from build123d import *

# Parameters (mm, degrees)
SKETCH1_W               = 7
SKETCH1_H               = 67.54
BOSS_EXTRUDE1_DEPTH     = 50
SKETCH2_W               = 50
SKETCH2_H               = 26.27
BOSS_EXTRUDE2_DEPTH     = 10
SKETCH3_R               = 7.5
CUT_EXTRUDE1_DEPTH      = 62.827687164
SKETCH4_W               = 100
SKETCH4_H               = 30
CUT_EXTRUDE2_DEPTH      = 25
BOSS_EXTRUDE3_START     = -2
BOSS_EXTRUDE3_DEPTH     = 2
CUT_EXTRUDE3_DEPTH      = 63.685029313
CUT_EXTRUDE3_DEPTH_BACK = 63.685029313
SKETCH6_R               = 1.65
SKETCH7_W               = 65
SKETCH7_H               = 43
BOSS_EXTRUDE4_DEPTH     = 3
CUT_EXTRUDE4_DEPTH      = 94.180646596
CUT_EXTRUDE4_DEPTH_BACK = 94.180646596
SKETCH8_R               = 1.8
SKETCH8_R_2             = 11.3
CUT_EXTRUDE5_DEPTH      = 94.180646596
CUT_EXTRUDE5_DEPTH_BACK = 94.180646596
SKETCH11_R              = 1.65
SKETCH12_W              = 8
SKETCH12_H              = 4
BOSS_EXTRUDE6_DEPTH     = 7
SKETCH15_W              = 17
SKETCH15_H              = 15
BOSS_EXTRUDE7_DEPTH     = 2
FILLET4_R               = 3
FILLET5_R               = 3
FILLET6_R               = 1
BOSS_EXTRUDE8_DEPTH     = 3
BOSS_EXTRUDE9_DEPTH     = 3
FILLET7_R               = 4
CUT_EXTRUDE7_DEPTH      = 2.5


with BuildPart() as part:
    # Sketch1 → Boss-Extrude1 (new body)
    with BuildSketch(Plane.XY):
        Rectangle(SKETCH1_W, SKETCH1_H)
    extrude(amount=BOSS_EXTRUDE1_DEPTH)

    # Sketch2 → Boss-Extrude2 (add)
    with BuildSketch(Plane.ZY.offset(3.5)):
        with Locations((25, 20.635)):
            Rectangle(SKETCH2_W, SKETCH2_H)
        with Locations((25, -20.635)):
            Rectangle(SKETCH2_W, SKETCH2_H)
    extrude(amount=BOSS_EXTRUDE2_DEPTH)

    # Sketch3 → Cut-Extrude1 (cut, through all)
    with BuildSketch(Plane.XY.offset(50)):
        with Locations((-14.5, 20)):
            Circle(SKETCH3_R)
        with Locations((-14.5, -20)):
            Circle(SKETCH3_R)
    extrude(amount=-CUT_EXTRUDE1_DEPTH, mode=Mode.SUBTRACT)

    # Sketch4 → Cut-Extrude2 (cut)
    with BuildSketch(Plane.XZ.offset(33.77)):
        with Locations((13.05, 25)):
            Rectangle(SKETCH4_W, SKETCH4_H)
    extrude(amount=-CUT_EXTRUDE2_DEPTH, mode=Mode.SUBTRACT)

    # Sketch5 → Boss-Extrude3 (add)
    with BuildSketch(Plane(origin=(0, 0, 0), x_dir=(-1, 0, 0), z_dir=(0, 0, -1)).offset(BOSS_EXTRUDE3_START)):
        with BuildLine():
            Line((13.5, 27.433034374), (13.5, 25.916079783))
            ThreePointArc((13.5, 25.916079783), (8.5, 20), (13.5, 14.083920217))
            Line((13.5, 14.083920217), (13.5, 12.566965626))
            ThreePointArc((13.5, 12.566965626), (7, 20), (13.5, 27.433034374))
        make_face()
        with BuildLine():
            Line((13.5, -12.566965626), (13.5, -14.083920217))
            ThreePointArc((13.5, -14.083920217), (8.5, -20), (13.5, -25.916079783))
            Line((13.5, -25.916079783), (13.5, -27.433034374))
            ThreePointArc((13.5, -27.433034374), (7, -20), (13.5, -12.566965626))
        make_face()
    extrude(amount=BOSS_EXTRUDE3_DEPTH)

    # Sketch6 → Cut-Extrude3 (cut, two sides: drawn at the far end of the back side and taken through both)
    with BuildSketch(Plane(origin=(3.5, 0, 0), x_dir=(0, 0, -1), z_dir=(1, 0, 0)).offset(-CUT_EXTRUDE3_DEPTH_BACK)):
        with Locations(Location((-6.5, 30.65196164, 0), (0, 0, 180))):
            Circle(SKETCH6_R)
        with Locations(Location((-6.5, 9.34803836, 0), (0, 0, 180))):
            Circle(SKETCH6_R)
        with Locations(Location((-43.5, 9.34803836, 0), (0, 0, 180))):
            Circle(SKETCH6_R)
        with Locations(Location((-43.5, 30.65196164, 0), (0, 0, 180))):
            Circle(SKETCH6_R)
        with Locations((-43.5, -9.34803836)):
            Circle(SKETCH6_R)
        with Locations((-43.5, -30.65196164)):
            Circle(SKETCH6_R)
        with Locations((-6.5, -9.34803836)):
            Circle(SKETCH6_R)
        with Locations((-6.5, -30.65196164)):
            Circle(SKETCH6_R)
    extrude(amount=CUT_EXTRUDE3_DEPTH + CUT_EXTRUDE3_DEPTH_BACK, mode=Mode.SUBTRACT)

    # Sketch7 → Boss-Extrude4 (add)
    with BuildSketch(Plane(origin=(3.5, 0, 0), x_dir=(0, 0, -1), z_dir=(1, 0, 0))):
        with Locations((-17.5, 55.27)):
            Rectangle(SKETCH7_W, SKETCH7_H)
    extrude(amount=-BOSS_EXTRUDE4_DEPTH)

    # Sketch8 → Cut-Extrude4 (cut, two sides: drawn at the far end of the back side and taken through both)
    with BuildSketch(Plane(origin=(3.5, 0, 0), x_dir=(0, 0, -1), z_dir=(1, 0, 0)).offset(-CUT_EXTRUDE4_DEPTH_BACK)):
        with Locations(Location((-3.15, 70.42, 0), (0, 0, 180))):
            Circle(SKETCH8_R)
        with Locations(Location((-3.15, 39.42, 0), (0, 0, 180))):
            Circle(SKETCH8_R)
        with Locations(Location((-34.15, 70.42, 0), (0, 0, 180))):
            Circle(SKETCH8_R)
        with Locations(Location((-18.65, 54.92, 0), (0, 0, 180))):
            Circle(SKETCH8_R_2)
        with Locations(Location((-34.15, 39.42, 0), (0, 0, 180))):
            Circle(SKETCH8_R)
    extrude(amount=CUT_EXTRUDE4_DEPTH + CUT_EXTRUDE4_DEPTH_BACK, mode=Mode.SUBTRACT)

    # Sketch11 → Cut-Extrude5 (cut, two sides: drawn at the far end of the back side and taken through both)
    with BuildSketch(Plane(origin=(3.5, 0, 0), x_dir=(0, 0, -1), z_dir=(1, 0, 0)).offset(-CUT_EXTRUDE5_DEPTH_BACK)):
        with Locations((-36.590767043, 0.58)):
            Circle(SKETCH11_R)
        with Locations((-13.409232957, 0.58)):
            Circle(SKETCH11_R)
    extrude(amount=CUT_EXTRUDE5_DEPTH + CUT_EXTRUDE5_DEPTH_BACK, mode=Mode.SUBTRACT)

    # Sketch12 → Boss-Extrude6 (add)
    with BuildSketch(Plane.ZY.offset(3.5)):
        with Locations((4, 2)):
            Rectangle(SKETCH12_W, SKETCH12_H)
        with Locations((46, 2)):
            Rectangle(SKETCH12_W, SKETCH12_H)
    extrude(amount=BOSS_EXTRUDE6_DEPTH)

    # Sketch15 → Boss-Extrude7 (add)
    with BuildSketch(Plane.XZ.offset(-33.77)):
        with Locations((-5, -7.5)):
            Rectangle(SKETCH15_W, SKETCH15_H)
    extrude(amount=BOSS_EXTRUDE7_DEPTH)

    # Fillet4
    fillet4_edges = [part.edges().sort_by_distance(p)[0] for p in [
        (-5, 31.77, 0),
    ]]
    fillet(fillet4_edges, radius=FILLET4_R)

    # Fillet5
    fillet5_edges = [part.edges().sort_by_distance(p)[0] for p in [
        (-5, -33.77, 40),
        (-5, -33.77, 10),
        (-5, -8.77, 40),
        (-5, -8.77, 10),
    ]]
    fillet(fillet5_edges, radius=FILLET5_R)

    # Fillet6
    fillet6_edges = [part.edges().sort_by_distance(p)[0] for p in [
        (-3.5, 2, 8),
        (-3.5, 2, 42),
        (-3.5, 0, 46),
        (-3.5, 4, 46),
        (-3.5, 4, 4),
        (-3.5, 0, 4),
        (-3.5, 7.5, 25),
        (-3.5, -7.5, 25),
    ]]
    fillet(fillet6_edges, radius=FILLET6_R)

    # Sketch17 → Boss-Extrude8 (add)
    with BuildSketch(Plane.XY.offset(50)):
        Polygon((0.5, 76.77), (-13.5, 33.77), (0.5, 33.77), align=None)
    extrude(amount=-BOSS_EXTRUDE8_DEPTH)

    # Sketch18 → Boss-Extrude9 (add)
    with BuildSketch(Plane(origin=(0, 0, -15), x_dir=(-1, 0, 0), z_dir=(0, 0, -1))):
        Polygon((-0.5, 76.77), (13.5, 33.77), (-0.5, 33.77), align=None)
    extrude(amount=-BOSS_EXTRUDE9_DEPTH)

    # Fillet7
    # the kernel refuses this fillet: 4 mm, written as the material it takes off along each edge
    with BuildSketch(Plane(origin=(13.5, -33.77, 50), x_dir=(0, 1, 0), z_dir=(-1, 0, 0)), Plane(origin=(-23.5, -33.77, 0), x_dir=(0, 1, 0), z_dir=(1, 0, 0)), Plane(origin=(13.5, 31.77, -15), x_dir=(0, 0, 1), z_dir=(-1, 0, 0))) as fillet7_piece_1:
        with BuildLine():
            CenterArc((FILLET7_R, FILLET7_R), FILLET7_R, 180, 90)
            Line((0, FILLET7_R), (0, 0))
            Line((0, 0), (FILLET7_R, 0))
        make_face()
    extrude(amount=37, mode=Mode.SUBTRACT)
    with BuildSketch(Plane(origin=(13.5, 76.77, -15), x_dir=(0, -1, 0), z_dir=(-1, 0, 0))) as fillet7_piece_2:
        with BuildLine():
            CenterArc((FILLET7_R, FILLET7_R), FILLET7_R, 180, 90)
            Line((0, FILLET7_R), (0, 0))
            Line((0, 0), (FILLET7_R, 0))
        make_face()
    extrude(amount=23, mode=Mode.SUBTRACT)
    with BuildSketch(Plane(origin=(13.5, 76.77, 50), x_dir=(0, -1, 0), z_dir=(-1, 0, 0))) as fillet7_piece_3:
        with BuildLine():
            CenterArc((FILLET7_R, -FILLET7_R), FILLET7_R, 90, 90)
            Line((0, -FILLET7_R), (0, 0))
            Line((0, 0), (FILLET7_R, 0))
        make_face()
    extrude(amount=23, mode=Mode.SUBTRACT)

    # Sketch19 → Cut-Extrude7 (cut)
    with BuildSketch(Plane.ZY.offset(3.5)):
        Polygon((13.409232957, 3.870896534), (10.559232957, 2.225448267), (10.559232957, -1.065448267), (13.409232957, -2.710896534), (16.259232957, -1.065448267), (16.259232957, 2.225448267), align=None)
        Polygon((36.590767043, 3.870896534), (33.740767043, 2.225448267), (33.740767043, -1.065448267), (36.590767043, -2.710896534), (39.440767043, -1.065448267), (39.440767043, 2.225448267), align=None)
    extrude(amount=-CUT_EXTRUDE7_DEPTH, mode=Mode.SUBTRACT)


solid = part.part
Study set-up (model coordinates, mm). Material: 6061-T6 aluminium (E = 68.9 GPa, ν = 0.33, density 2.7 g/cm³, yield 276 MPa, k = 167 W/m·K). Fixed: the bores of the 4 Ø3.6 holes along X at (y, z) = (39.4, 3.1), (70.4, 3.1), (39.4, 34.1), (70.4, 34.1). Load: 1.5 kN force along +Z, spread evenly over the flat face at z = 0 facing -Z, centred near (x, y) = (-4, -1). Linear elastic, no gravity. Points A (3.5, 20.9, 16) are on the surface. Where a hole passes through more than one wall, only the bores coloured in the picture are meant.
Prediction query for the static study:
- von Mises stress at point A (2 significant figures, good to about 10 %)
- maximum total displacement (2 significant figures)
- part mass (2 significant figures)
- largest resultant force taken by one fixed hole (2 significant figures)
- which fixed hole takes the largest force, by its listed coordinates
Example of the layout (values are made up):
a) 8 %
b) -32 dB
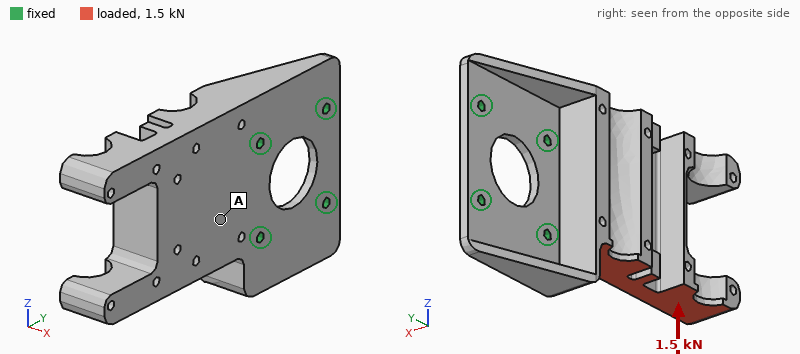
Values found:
a) 7.2 MPa
b) 94 µm
c) 110 g
d) 1.7 kN
e) (39.4, 3.1)
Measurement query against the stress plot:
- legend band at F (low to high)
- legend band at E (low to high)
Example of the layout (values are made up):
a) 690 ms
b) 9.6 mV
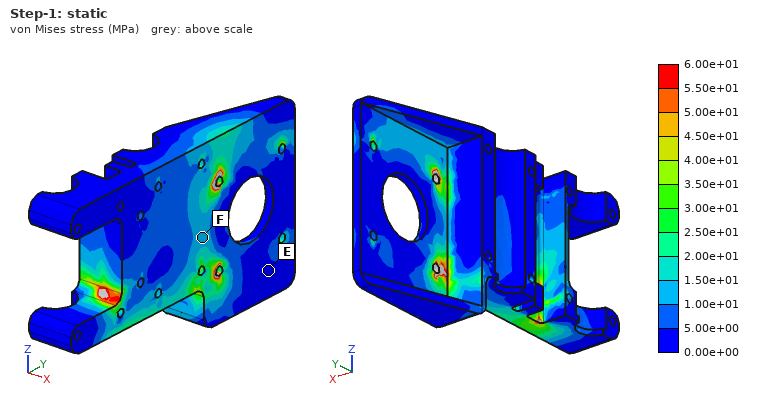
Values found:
a) 1.00e+01 to 1.50e+01 MPa
b) 0.00e+00 to 5.00e+00 MPa
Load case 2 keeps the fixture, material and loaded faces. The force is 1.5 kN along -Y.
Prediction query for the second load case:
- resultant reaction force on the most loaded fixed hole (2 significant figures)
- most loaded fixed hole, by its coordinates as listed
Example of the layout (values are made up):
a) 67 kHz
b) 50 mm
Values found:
a) 1.5 kN
b) (39.4, 3.1)
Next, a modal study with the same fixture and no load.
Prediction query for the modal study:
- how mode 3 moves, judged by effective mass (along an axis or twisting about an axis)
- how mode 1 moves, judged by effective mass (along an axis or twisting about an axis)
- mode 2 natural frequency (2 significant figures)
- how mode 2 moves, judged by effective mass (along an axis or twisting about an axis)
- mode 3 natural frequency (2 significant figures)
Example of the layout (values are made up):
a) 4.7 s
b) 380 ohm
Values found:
a) along Z
b) along X
c) 2400 Hz
d) twisting about Y
e) 4100 Hz
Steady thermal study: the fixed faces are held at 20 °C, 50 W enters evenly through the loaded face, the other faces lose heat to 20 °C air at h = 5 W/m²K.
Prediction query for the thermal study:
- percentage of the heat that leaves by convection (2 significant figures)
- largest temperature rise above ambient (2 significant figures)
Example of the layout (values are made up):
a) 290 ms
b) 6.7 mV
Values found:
a) 4.1 %
b) 65 K
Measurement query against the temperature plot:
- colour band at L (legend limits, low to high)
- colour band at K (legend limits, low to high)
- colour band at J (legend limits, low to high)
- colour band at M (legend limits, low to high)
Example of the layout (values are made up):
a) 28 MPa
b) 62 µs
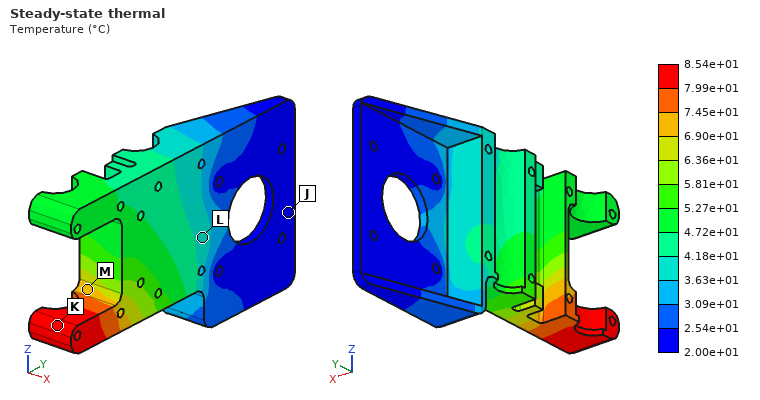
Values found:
a) 3.63e+01 to 4.18e+01 °C
b) 7.99e+01 to 8.54e+01 °C
c) 2.00e+01 to 2.54e+01 °C
d) 6.90e+01 to 7.45e+01 °C
